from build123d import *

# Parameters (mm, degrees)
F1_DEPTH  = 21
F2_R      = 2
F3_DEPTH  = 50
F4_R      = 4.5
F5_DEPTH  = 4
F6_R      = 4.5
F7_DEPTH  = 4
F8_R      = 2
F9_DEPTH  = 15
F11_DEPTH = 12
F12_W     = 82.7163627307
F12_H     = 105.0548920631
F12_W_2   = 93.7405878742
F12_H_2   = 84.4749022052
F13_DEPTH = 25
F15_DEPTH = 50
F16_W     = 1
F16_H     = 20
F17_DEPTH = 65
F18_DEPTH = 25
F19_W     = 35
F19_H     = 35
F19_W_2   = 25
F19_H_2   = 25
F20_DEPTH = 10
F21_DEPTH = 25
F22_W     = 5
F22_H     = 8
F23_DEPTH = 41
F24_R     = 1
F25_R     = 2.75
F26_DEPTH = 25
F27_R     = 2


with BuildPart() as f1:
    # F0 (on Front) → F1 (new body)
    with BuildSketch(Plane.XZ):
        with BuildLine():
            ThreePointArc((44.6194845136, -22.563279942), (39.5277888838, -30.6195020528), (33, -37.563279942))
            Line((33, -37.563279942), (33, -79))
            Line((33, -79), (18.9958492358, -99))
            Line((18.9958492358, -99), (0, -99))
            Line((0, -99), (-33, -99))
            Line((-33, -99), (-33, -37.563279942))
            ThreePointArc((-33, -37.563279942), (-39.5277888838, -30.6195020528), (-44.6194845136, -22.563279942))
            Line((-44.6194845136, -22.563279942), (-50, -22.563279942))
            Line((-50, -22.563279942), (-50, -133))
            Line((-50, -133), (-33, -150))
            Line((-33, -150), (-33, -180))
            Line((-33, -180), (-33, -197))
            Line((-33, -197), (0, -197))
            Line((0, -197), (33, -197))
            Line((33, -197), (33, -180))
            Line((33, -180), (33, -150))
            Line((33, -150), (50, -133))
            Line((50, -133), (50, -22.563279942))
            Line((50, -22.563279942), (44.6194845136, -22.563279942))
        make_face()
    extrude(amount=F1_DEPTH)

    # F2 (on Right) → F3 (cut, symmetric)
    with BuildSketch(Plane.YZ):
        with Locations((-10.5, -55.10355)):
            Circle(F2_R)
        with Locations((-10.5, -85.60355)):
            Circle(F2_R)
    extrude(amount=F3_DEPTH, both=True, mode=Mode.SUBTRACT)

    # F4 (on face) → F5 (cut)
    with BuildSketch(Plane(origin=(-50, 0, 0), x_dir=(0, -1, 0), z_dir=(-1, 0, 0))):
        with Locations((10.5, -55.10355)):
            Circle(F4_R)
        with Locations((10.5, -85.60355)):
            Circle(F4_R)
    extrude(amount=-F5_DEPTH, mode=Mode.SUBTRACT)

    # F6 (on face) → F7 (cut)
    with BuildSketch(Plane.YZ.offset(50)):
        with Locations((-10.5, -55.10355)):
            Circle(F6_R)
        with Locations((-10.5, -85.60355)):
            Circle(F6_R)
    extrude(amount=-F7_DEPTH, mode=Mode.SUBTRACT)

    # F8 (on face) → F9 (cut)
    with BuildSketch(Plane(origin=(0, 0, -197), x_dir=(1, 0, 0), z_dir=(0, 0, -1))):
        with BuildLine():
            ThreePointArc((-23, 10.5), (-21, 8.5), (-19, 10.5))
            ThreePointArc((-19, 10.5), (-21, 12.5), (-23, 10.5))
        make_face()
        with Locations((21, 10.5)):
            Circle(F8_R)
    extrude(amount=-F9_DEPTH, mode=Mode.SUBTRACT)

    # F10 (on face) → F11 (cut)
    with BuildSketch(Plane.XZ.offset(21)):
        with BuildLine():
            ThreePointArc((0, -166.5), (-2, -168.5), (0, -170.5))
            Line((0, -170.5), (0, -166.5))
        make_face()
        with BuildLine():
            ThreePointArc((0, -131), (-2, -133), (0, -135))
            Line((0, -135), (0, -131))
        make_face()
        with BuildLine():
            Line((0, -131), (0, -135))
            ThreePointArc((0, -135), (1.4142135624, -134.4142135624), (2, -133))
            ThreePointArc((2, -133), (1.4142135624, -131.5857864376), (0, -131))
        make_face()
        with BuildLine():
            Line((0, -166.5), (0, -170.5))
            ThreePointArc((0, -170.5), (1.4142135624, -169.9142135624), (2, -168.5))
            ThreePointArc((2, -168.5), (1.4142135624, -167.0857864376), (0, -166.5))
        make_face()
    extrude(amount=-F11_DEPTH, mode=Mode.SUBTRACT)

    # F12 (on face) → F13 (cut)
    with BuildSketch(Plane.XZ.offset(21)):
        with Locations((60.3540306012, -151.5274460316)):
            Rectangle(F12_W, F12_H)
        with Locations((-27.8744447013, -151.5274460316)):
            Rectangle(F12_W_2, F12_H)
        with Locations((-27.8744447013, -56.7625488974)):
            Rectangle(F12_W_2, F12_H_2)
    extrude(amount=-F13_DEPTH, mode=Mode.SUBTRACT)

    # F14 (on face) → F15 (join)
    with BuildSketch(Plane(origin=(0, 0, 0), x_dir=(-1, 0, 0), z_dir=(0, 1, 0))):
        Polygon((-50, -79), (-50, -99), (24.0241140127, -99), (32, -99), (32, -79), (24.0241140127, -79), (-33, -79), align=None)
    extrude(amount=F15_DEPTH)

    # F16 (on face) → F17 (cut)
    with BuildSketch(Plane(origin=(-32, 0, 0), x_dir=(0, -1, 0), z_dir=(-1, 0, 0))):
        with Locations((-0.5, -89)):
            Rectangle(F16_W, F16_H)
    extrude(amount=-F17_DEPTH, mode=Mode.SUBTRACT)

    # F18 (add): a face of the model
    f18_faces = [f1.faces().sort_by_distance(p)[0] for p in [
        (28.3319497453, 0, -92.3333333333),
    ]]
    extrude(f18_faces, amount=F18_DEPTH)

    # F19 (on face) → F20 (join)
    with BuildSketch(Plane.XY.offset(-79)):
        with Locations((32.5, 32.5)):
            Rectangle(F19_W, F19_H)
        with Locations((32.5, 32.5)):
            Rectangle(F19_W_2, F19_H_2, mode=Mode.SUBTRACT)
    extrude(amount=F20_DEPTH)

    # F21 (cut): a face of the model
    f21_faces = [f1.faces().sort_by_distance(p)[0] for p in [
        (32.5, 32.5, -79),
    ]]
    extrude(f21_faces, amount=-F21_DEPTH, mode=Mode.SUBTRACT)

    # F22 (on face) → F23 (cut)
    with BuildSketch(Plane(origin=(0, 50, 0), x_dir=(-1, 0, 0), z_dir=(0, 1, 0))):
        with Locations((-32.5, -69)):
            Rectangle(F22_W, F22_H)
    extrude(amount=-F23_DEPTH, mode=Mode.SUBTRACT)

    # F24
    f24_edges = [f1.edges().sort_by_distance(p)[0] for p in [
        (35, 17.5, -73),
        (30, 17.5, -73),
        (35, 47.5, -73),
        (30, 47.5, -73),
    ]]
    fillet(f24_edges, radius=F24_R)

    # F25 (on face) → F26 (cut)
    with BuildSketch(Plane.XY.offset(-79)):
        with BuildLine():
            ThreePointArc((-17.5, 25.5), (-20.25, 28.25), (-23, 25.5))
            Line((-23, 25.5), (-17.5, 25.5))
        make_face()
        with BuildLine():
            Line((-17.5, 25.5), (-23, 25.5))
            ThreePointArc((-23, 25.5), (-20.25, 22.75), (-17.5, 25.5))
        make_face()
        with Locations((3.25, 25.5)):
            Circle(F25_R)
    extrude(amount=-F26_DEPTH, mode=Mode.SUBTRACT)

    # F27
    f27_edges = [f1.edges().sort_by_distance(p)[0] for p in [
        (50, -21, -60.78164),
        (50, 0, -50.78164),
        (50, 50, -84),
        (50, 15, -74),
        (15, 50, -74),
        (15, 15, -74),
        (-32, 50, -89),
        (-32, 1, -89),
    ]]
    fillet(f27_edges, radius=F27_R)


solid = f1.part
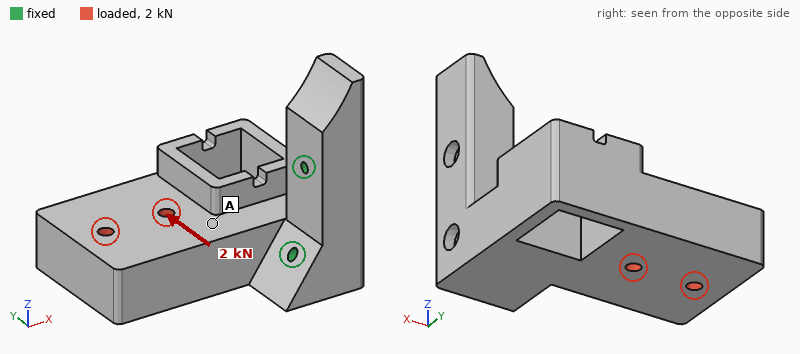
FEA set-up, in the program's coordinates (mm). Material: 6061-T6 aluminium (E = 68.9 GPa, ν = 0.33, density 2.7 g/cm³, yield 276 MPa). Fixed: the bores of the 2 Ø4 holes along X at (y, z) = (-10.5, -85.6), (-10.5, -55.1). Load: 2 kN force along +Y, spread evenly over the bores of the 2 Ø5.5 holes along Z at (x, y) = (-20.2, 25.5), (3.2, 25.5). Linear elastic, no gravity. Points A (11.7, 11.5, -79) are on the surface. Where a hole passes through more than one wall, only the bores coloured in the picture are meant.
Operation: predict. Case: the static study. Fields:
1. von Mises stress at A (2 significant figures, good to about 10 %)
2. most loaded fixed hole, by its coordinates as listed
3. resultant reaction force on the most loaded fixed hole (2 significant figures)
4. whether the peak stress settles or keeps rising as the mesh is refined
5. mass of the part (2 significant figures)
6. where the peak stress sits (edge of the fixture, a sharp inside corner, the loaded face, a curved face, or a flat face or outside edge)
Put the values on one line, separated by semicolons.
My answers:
15 MPa; (-10.5, -85.6); 2.2 kN; keeps rising; 270 g; edge of the fixture
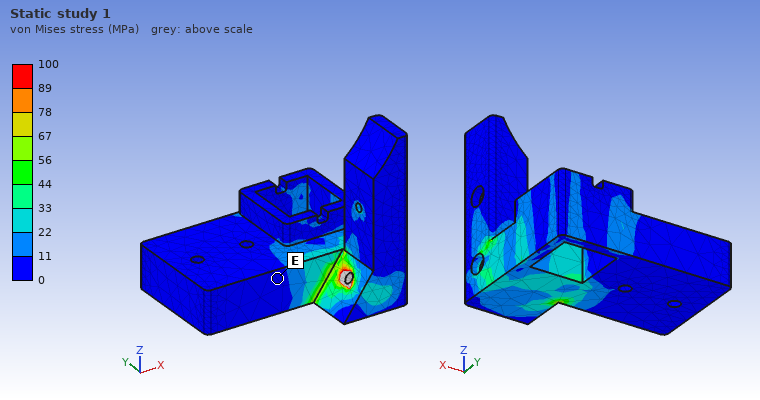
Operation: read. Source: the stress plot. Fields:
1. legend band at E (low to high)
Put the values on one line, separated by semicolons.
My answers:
0 to 11 MPa
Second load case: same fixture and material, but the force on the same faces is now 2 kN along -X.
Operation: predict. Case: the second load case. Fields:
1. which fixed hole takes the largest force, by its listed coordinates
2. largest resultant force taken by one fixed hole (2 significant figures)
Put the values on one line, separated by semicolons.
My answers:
(-10.5, -85.6); 2.0 kN
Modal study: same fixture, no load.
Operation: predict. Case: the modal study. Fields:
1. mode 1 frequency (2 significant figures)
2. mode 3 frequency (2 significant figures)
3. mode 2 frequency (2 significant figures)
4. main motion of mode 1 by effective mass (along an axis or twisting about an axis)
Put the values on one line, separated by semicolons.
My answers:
1200 Hz; 3000 Hz; 1400 Hz; along Z
